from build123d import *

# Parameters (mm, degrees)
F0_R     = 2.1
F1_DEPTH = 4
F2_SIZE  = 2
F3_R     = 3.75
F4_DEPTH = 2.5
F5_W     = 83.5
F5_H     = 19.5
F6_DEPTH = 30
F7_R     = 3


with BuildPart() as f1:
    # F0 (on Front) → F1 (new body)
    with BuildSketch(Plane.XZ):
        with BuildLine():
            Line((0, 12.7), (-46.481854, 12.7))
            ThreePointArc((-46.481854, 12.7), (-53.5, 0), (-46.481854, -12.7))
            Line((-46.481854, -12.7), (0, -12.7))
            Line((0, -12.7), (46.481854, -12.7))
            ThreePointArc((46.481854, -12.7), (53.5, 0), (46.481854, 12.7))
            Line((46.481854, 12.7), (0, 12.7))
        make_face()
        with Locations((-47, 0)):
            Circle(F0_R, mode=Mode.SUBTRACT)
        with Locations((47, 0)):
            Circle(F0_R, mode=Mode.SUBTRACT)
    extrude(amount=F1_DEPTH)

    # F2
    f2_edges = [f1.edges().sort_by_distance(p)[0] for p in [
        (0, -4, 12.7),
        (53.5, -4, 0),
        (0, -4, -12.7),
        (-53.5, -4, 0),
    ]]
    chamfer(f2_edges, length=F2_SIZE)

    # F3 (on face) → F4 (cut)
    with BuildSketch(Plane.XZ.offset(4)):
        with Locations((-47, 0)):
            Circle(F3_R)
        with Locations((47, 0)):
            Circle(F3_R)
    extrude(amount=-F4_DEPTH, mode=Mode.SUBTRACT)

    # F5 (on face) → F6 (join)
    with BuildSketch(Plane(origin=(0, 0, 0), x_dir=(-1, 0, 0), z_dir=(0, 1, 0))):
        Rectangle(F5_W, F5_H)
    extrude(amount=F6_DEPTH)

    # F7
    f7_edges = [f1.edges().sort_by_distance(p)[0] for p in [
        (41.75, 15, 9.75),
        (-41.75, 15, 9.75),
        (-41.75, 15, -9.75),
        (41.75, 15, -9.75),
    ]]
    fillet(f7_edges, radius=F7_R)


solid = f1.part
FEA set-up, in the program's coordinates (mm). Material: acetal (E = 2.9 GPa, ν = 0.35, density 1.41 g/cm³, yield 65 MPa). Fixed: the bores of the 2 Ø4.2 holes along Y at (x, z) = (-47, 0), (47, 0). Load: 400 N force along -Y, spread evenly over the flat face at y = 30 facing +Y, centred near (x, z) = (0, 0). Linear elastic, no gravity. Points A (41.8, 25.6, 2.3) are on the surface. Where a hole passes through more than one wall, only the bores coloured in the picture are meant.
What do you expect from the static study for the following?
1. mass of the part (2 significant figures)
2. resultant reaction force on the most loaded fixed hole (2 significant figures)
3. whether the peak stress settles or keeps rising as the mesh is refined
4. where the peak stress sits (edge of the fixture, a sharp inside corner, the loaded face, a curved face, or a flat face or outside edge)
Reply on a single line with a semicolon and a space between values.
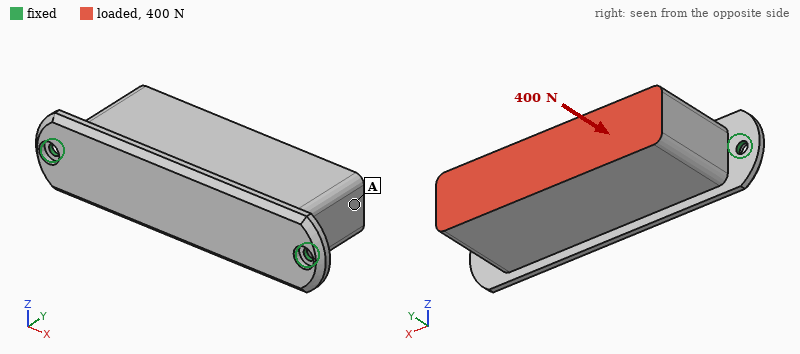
82 g; 200 N; keeps rising; edge of the fixture
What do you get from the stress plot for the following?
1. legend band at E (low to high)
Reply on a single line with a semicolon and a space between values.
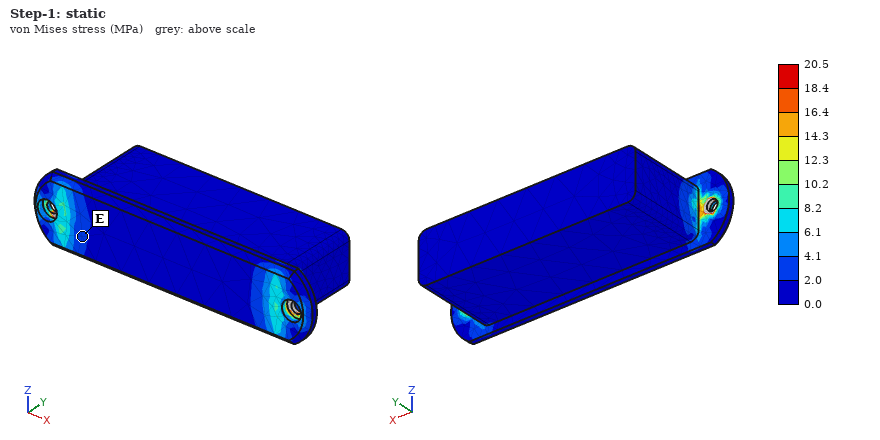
2.0 to 4.1 MPa
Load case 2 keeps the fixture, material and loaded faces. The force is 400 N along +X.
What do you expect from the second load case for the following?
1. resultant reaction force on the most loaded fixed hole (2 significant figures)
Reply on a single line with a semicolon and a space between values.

240 N
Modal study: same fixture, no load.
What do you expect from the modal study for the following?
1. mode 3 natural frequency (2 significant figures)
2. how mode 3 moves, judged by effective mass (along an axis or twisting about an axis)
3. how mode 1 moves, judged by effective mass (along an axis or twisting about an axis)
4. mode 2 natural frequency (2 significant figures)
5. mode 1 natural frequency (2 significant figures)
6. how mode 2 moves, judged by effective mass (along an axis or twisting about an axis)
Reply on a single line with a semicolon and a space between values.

1500 Hz; along X; along Z; 1000 Hz; 220 Hz; along Y
